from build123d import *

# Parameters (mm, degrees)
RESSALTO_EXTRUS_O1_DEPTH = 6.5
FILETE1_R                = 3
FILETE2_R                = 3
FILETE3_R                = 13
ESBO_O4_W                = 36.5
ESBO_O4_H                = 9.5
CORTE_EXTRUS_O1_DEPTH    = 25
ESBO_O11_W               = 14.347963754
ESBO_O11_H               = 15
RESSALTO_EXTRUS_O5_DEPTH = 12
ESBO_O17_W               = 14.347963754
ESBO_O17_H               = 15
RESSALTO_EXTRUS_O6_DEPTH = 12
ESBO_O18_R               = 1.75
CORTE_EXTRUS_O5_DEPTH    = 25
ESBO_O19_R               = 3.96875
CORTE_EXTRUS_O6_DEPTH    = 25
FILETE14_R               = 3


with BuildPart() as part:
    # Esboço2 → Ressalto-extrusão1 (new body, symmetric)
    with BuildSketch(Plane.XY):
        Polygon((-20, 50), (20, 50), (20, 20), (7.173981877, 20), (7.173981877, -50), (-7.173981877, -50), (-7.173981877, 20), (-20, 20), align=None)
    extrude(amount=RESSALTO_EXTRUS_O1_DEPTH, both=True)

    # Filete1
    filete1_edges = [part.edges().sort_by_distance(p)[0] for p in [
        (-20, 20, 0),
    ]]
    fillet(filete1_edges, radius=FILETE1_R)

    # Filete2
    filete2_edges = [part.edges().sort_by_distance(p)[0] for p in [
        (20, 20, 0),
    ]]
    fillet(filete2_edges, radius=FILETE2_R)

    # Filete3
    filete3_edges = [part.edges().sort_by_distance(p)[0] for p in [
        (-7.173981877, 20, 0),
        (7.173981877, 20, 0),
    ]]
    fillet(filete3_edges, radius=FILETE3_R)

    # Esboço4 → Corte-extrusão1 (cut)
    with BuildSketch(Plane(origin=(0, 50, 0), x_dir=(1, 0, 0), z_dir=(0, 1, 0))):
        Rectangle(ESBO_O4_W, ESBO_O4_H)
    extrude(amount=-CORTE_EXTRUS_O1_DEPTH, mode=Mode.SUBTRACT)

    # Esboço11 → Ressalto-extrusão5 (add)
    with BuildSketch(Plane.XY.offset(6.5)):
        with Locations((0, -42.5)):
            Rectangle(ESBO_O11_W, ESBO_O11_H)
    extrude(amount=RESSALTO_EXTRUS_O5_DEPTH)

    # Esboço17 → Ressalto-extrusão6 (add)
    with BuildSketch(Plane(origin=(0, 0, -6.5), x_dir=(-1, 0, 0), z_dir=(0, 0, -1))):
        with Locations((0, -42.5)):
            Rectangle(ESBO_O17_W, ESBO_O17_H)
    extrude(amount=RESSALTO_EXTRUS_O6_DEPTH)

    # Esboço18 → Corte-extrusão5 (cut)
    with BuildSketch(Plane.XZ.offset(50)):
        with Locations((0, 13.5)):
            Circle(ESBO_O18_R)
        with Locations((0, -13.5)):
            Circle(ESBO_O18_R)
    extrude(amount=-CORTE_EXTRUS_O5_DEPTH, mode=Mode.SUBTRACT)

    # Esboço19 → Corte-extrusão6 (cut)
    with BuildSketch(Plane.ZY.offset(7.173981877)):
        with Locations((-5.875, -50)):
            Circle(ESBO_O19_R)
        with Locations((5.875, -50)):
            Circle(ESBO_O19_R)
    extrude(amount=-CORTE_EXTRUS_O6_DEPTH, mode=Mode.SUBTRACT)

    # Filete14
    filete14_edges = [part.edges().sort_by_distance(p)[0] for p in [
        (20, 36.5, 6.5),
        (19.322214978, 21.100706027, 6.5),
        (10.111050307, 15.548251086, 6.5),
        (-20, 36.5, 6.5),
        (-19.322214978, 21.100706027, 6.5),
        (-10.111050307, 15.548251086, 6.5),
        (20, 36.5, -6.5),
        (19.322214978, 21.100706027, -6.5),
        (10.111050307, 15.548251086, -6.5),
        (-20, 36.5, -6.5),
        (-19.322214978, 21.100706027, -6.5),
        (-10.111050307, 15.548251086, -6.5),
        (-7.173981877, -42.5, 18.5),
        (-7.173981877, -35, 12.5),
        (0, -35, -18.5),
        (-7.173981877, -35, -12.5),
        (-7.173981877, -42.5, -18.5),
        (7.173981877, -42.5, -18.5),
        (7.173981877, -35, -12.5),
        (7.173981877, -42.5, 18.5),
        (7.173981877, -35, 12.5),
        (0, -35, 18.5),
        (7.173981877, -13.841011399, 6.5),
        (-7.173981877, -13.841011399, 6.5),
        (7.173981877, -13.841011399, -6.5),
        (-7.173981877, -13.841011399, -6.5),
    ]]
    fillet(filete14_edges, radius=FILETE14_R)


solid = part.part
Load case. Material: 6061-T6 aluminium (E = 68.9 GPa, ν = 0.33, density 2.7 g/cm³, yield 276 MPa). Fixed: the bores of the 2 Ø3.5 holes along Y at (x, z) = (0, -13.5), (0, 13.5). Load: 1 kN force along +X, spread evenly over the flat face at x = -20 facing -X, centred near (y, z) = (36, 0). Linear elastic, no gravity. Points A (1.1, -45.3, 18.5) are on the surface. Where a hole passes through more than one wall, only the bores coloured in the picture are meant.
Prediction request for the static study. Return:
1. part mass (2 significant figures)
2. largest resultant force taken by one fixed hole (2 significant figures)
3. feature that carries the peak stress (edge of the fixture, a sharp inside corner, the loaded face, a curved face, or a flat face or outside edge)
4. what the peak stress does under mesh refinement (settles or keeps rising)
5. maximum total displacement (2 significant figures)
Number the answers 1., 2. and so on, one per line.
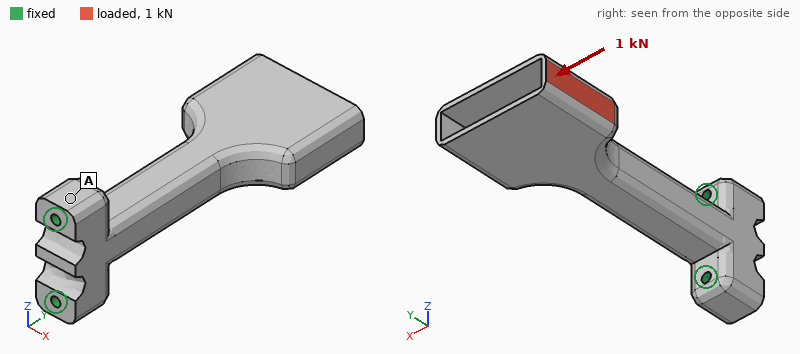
1. 65 g
2. 500 N
3. edge of the fixture
4. keeps rising
5. 1.3 mm
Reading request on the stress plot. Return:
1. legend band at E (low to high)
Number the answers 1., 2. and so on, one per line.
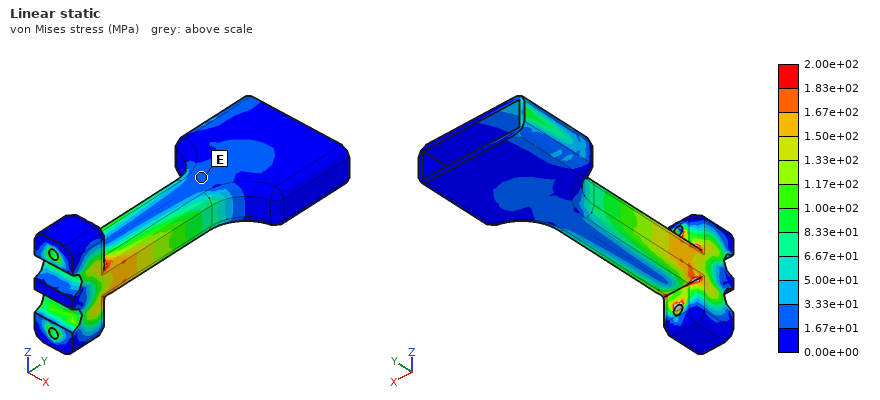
1. 1.67e+01 to 3.33e+01 MPa
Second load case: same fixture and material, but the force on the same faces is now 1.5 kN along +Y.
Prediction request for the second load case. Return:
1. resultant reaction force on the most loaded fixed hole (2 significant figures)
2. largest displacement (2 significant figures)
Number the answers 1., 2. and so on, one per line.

1. 780 N
2. 0.68 mm
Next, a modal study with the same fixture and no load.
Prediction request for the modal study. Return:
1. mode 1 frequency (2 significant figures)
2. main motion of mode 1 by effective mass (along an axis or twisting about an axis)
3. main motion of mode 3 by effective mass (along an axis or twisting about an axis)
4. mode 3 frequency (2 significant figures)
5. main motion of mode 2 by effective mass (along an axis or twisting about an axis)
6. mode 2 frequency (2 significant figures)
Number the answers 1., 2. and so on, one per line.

1. 1100 Hz
2. along X
3. twisting about Y
4. 3700 Hz
5. along Z
6. 1200 Hz
